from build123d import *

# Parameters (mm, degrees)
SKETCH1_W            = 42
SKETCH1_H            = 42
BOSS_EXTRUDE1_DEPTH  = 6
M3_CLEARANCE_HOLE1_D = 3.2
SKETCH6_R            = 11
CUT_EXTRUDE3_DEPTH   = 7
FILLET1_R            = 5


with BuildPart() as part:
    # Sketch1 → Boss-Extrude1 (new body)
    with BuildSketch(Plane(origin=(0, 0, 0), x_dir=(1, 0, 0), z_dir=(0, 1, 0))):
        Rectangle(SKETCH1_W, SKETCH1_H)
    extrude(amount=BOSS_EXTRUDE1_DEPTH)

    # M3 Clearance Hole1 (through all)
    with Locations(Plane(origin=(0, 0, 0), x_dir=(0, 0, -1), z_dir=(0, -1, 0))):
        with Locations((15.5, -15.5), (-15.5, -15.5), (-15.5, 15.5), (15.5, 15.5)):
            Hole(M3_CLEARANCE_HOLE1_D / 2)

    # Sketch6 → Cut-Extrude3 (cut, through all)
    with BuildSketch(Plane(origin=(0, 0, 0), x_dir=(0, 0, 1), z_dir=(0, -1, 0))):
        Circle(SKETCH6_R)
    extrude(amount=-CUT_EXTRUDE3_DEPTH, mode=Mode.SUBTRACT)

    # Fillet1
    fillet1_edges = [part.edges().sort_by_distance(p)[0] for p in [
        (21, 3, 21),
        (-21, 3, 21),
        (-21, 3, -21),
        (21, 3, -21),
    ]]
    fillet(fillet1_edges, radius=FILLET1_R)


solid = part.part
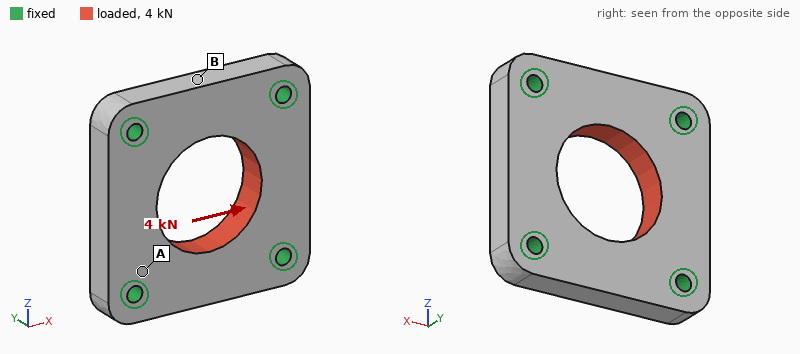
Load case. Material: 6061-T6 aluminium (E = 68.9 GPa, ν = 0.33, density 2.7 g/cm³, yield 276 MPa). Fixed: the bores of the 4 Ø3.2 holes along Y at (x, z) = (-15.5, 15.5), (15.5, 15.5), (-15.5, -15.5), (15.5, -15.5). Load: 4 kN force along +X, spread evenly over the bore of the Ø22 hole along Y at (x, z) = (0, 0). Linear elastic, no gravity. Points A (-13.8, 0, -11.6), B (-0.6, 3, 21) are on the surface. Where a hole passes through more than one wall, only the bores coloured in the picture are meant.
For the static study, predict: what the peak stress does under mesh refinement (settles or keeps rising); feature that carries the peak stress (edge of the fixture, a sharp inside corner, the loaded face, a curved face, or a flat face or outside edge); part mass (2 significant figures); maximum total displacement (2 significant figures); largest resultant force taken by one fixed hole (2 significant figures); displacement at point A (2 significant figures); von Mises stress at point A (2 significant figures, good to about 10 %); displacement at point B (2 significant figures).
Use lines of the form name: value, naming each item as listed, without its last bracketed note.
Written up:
what the peak stress does under mesh refinement: keeps rising
feature that carries the peak stress: edge of the fixture
part mass: 22 g
maximum total displacement: 6.3 µm
largest resultant force taken by one fixed hole: 1.0 kN
displacement at point A: 1.8 µm
von Mises stress at point A: 16 MPa
displacement at point B: 1.5 µm
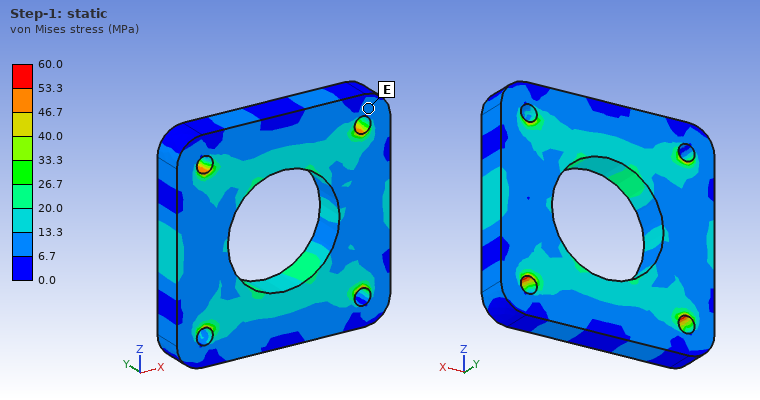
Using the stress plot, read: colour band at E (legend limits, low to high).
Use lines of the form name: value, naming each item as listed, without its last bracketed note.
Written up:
colour band at E: 6.7 to 13.3 MPa
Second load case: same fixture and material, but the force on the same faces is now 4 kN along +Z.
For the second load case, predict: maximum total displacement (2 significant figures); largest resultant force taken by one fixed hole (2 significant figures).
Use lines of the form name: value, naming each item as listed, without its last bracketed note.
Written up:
maximum total displacement: 6.3 µm
largest resultant force taken by one fixed hole: 1.0 kN
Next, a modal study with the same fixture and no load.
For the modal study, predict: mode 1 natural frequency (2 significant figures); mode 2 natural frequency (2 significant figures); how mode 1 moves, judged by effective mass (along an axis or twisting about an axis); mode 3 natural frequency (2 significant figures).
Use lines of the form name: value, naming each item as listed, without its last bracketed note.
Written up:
mode 1 natural frequency: 25 kHz
mode 2 natural frequency: 28 kHz
how mode 1 moves, judged by effective mass: along Y
mode 3 natural frequency: 28 kHz
